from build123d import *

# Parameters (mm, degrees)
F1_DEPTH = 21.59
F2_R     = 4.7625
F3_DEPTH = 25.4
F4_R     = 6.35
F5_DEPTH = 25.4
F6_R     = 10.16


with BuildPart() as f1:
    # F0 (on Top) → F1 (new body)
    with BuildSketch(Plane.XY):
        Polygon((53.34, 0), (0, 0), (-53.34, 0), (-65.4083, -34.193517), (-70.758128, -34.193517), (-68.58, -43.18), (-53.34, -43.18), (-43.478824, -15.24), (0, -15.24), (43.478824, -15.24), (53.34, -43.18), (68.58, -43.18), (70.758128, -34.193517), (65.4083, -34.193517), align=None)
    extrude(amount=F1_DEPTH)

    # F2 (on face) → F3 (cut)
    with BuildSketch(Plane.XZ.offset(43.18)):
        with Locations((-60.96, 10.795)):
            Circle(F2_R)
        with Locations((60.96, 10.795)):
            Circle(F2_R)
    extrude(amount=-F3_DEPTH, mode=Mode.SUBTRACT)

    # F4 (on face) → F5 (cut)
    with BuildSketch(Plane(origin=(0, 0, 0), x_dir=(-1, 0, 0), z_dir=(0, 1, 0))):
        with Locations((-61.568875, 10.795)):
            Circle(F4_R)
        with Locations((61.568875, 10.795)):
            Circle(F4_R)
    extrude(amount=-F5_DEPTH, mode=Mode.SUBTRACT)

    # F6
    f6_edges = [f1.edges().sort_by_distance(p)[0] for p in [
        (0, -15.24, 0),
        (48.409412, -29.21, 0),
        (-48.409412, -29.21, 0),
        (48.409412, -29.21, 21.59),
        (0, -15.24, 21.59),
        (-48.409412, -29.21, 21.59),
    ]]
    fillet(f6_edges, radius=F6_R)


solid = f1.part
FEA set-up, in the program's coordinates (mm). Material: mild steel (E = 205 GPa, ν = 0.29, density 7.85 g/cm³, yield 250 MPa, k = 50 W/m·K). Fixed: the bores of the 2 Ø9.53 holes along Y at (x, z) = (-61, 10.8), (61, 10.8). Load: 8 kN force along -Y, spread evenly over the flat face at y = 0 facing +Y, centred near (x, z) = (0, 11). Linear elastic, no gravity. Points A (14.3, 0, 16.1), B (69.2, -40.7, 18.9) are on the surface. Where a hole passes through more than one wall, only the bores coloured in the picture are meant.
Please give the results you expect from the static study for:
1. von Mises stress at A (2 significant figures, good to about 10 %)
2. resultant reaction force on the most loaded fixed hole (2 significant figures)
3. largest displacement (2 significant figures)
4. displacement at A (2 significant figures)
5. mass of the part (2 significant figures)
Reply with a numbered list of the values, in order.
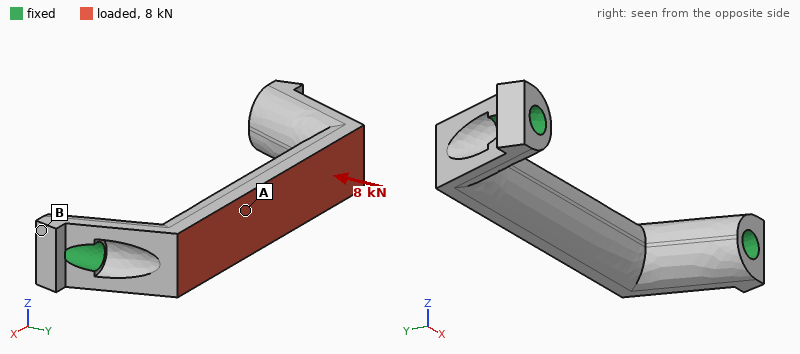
1. 56 MPa
2. 5.4 kN
3. 37 µm
4. 32 µm
5. 360 g
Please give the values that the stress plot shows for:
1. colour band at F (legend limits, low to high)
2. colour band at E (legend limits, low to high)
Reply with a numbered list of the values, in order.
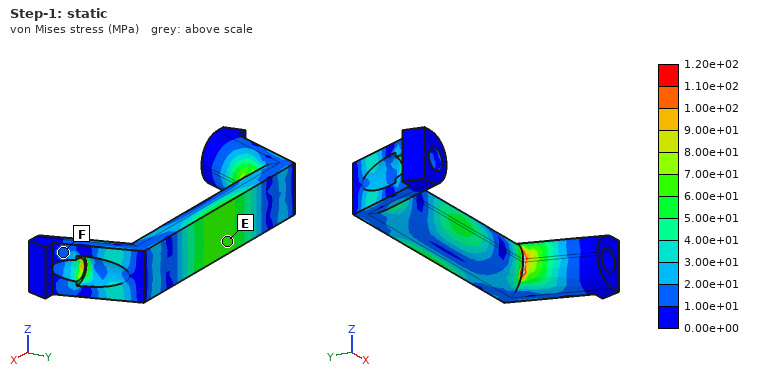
1. 1.00e+01 to 2.00e+01 MPa
2. 6.00e+01 to 7.00e+01 MPa
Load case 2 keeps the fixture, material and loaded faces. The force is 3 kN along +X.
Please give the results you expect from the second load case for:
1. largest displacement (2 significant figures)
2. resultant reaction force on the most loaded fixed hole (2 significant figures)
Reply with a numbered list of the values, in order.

1. 8.2 µm
2. 1.6 kN
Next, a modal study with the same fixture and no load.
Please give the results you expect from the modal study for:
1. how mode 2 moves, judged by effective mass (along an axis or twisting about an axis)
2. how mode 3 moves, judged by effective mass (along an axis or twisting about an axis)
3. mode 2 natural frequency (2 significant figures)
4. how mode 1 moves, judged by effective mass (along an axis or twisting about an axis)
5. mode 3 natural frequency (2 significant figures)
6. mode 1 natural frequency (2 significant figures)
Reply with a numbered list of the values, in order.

1. along Y
2. along X
3. 5400 Hz
4. along Z
5. 6000 Hz
6. 4000 Hz
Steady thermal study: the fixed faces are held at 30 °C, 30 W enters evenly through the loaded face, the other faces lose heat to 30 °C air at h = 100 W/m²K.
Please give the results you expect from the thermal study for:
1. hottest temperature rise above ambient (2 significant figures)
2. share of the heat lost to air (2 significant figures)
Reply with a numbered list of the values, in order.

1. 32 K
2. 46 %
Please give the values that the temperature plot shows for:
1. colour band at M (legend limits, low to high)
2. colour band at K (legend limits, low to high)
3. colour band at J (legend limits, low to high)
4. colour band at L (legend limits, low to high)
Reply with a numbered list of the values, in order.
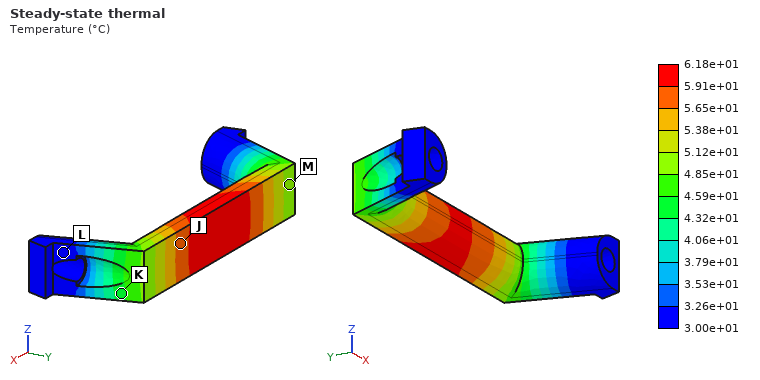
1. 4.85e+01 to 5.12e+01 °C
2. 4.32e+01 to 4.59e+01 °C
3. 5.65e+01 to 5.91e+01 °C
4. 3.00e+01 to 3.26e+01 °C
